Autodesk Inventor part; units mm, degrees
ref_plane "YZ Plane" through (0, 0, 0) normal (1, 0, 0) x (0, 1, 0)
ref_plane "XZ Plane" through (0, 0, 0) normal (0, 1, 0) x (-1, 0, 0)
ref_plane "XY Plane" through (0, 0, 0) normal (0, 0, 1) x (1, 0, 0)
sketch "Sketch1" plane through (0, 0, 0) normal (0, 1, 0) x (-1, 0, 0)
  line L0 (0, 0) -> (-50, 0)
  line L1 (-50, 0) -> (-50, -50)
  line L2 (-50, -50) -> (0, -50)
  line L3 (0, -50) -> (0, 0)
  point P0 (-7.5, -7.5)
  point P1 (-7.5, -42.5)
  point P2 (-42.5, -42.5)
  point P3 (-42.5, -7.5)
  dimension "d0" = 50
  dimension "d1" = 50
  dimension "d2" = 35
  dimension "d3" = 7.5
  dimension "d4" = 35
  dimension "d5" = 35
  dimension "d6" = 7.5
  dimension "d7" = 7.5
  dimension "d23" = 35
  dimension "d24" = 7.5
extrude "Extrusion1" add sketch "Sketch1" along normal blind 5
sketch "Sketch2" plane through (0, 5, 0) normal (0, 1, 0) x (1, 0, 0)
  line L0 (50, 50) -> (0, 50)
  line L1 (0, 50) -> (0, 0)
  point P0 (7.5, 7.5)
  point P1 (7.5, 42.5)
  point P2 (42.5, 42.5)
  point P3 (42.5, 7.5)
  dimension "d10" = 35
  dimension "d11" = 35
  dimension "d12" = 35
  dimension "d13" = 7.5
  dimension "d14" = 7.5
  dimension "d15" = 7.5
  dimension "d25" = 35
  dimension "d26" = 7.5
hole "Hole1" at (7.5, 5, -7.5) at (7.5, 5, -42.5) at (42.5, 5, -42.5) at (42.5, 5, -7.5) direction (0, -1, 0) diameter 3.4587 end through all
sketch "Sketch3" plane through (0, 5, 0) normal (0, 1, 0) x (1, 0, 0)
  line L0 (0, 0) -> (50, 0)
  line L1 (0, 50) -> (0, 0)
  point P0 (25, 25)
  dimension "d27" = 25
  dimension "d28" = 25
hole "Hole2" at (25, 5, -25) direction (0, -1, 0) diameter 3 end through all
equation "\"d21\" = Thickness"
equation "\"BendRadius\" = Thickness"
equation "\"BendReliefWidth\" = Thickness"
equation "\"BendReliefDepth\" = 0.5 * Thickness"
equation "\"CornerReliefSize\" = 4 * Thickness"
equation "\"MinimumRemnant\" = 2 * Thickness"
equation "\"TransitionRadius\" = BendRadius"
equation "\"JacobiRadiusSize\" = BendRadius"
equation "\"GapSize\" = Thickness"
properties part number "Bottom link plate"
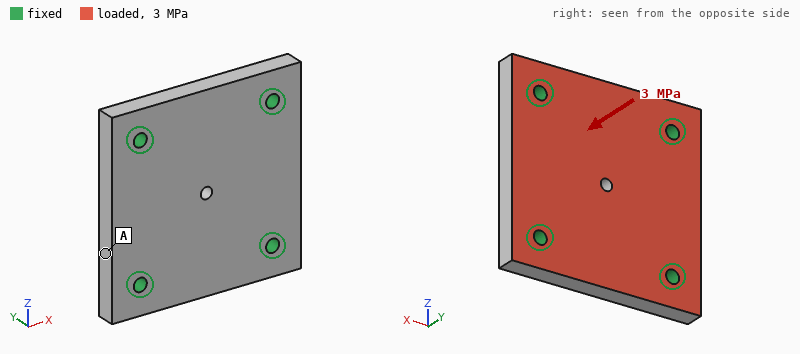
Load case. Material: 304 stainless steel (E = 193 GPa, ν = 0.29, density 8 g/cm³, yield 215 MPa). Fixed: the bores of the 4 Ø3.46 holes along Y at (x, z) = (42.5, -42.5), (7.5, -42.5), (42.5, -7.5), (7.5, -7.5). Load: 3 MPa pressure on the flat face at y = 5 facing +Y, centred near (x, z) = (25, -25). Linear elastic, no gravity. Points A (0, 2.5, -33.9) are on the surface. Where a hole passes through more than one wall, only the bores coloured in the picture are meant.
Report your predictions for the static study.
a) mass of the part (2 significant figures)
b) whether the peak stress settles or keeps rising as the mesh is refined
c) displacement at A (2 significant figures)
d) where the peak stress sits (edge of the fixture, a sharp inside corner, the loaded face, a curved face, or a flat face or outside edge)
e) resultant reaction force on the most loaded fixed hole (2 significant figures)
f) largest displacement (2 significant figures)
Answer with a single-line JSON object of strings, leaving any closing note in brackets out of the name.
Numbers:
{"mass of the part": "98 g", "whether the peak stress settles or keeps rising as the mesh is refined": "keeps rising", "displacement at A": "3.9 µm", "where the peak stress sits": "edge of the fixture", "resultant reaction force on the most loaded fixed hole": "1.8 kN", "largest displacement": "16 µm"}
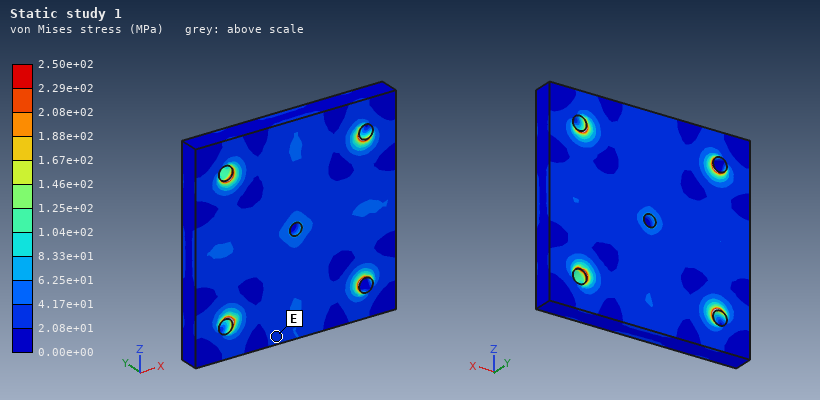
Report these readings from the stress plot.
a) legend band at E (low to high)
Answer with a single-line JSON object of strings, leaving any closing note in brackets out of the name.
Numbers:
{"legend band at E": "2.08e+01 to 4.17e+01 MPa"}
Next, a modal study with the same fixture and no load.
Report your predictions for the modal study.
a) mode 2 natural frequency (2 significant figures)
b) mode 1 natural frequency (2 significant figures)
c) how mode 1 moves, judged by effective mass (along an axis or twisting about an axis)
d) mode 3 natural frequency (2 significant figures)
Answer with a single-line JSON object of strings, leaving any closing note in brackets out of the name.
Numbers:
{"mode 2 natural frequency": "19 kHz", "mode 1 natural frequency": "13 kHz", "how mode 1 moves, judged by effective mass": "along Y", "mode 3 natural frequency": "19 kHz"}
